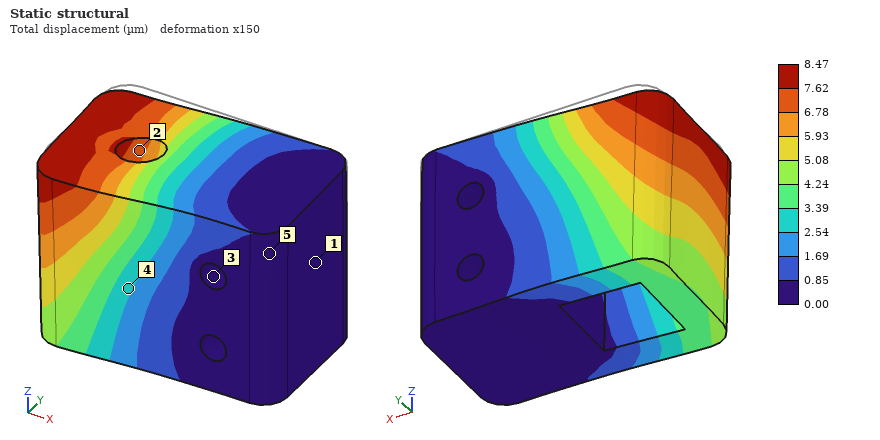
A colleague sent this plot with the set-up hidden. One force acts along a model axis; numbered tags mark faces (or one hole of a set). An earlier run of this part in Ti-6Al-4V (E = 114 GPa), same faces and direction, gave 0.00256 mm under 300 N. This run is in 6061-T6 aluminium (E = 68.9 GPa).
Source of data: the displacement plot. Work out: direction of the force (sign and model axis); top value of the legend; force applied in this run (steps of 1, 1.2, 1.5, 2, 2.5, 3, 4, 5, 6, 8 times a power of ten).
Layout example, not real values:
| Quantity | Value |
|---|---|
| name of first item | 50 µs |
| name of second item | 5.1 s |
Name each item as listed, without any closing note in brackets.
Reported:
| Quantity | Value |
|---|---|
| direction of the force | -Y |
| top value of the legend | 8.47 µm |
| force applied in this run | 600 N |
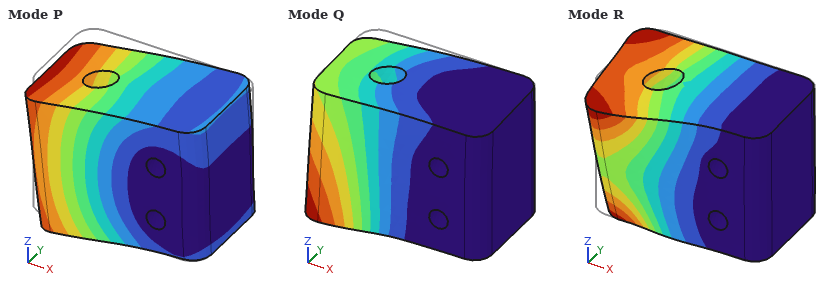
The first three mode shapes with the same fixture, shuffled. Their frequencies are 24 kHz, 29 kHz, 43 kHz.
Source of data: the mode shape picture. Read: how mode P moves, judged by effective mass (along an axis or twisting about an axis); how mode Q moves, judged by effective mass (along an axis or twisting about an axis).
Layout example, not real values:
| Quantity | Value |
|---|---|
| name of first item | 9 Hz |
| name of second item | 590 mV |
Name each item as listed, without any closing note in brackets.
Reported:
| Quantity | Value |
|---|---|
| how mode P moves, judged by effective mass | along Z |
| how mode Q moves, judged by effective mass | along Y |
